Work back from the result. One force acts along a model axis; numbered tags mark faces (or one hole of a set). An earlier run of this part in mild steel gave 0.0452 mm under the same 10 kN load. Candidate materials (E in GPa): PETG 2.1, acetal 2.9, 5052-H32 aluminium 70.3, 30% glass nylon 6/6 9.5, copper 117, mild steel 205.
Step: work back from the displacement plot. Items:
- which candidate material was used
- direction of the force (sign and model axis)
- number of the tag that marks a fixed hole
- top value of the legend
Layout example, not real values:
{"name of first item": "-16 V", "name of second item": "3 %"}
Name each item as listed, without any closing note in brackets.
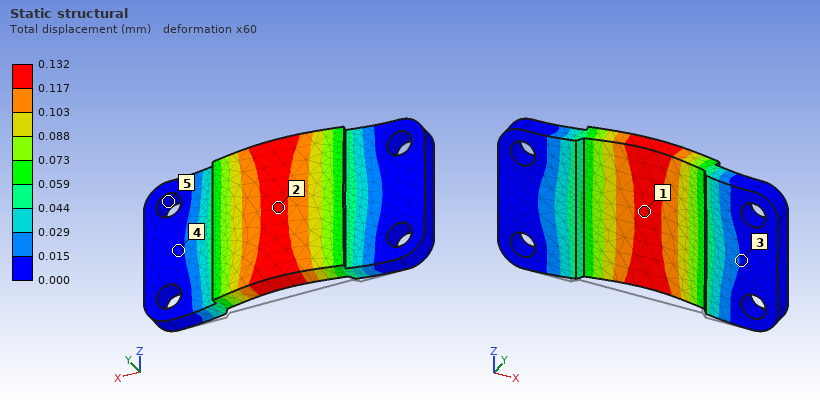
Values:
{"which candidate material was used": "5052-H32 aluminium", "direction of the force": "+Y", "number of the tag that marks a fixed hole": "5", "top value of the legend": "0.132 mm"}
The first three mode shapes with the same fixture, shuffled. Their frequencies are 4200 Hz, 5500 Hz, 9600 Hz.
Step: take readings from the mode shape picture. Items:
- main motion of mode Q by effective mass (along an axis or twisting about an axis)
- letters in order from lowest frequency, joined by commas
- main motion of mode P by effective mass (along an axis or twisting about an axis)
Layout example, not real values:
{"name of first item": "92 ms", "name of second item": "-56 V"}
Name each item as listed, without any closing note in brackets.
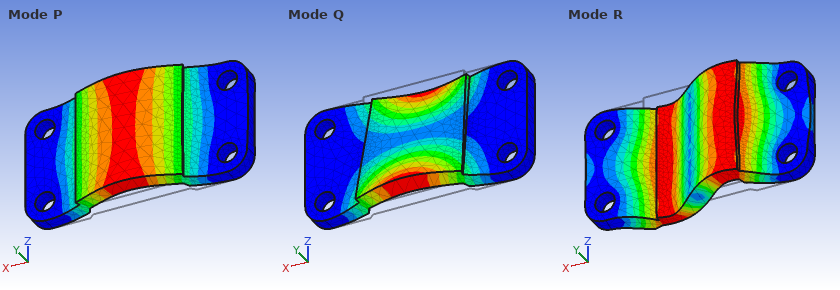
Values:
{"main motion of mode Q by effective mass": "twisting about X", "letters in order from lowest frequency, joined by commas": "P, Q, R", "main motion of mode P by effective mass": "along Y"}
